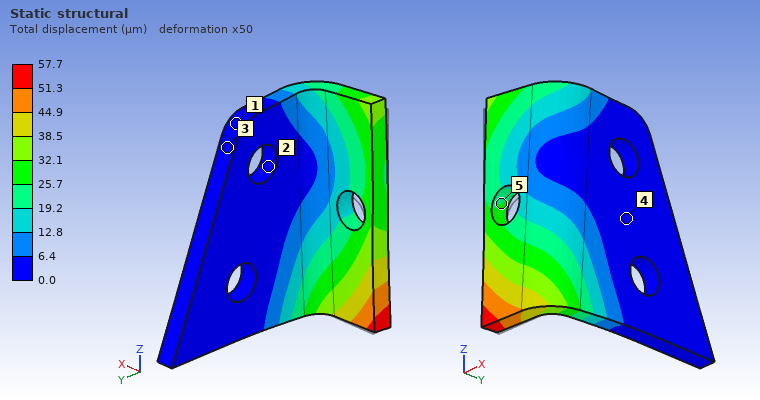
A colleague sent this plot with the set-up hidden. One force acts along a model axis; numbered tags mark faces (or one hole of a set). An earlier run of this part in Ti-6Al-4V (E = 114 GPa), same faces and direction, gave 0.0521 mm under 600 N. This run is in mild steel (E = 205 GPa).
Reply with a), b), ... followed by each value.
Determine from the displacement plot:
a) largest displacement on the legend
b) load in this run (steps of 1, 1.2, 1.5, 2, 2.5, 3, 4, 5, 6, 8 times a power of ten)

a) 57.7 µm
b) 1.2 kN
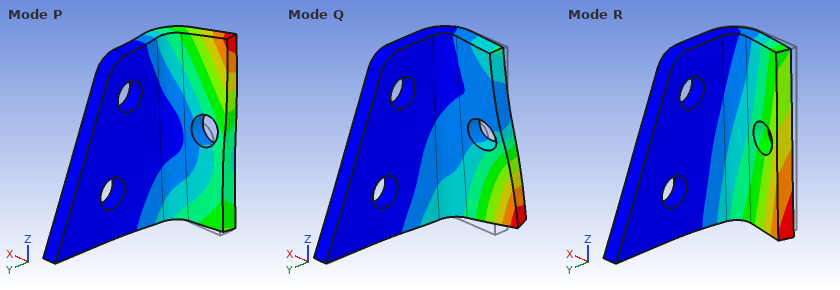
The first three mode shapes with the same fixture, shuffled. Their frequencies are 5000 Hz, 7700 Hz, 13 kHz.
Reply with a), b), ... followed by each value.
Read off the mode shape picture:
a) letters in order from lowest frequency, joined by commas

a) R, P, Q
